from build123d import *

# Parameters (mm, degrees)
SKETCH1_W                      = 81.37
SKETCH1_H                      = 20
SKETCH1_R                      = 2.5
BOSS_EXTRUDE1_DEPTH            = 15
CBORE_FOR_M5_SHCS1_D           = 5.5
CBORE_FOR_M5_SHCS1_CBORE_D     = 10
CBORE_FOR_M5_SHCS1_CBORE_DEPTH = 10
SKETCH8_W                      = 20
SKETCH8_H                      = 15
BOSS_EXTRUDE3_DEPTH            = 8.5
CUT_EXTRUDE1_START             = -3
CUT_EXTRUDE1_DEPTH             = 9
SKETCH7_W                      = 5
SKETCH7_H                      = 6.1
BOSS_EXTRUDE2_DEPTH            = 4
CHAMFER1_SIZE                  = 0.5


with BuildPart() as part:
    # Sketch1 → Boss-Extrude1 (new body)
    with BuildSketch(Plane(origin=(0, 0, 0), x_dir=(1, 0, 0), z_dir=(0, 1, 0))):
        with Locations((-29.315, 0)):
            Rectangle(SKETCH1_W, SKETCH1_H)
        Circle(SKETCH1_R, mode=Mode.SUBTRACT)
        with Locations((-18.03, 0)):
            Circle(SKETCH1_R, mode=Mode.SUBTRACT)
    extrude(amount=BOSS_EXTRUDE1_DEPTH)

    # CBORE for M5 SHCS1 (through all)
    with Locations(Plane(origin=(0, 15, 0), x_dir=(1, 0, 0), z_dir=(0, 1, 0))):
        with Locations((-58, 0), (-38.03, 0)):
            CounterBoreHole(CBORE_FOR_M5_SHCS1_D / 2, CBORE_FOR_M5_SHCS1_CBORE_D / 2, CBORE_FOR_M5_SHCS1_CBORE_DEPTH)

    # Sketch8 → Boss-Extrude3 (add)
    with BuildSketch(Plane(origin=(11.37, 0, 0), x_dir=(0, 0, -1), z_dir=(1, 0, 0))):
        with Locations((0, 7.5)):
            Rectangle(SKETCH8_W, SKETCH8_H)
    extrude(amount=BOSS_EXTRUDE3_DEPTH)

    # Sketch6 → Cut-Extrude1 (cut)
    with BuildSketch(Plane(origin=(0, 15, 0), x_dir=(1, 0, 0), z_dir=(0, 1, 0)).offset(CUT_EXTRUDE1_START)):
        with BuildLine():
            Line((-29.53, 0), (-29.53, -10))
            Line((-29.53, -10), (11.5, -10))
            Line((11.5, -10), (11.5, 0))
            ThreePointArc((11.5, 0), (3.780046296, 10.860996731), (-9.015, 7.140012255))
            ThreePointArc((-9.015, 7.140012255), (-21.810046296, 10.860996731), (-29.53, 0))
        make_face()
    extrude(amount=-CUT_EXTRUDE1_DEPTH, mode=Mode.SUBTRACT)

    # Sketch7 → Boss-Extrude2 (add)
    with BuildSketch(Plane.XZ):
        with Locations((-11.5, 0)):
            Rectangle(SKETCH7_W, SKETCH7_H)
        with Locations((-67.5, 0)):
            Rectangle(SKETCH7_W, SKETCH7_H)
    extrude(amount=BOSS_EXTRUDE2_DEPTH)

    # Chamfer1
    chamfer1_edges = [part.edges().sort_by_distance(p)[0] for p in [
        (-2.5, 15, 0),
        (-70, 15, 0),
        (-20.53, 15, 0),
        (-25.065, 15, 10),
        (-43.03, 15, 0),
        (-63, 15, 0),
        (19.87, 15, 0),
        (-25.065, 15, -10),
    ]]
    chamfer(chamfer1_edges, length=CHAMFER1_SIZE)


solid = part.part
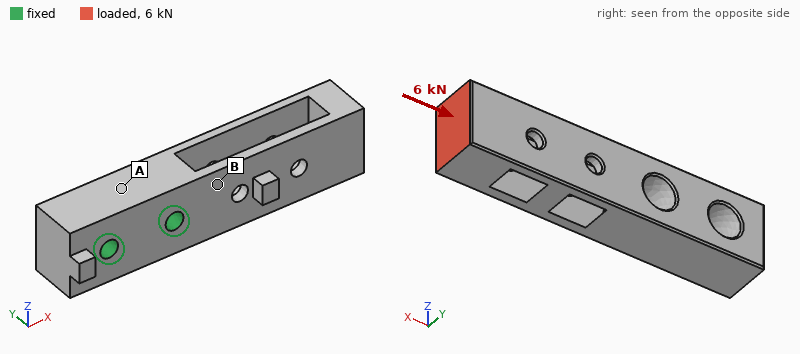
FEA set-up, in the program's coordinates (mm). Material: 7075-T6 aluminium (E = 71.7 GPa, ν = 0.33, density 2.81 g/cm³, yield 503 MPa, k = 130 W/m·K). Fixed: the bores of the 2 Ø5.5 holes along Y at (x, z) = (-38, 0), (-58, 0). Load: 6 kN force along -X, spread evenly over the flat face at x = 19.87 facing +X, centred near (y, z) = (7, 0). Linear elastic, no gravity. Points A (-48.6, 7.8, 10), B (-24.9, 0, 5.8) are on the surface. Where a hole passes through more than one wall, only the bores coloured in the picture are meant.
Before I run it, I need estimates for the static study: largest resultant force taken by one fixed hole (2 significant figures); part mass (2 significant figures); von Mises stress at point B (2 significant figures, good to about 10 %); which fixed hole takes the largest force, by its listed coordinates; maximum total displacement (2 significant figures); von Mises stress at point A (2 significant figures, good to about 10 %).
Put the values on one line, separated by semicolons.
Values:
4.2 kN; 51 g; 57 MPa; (-38, 0); 68 µm; 18 MPa
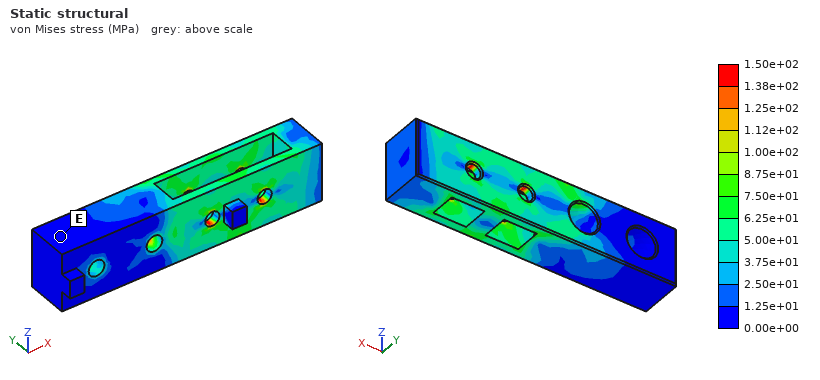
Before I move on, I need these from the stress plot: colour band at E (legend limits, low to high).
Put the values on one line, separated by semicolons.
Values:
0.00e+00 to 1.25e+01 MPa
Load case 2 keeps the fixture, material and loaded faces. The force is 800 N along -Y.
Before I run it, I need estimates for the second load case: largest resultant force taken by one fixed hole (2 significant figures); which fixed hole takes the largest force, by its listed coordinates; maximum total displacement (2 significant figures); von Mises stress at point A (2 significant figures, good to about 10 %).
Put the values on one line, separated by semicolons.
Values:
3.0 kN; (-38, 0); 0.79 mm; 23 MPa
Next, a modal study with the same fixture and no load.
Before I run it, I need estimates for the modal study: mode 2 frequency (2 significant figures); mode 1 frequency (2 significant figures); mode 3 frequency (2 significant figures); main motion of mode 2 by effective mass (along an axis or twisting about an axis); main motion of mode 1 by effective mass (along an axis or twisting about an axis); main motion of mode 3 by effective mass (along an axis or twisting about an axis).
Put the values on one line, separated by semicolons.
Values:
3200 Hz; 1600 Hz; 5500 Hz; along Z; along Y; twisting about X
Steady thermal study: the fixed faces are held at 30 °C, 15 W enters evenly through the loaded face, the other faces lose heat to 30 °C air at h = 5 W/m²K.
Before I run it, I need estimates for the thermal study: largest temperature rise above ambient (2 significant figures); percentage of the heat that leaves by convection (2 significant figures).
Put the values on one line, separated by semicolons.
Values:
52 K; 5.1 %
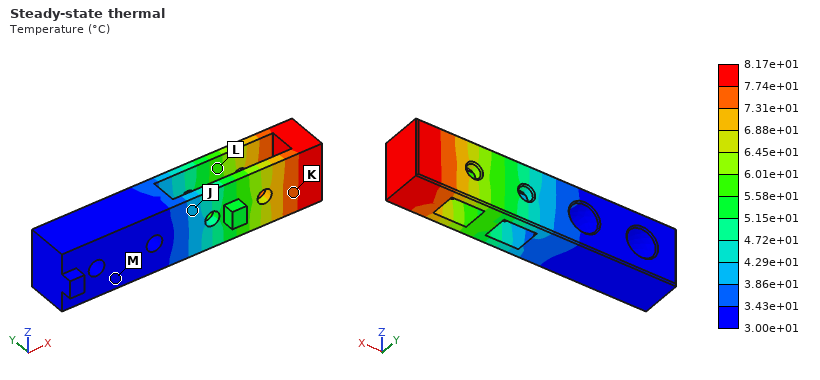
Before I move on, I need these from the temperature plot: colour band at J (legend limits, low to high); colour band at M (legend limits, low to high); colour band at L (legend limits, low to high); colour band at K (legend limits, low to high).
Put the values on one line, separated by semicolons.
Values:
3.86e+01 to 4.29e+01 °C; 3.00e+01 to 3.43e+01 °C; 5.58e+01 to 6.01e+01 °C; 7.31e+01 to 7.74e+01 °C
